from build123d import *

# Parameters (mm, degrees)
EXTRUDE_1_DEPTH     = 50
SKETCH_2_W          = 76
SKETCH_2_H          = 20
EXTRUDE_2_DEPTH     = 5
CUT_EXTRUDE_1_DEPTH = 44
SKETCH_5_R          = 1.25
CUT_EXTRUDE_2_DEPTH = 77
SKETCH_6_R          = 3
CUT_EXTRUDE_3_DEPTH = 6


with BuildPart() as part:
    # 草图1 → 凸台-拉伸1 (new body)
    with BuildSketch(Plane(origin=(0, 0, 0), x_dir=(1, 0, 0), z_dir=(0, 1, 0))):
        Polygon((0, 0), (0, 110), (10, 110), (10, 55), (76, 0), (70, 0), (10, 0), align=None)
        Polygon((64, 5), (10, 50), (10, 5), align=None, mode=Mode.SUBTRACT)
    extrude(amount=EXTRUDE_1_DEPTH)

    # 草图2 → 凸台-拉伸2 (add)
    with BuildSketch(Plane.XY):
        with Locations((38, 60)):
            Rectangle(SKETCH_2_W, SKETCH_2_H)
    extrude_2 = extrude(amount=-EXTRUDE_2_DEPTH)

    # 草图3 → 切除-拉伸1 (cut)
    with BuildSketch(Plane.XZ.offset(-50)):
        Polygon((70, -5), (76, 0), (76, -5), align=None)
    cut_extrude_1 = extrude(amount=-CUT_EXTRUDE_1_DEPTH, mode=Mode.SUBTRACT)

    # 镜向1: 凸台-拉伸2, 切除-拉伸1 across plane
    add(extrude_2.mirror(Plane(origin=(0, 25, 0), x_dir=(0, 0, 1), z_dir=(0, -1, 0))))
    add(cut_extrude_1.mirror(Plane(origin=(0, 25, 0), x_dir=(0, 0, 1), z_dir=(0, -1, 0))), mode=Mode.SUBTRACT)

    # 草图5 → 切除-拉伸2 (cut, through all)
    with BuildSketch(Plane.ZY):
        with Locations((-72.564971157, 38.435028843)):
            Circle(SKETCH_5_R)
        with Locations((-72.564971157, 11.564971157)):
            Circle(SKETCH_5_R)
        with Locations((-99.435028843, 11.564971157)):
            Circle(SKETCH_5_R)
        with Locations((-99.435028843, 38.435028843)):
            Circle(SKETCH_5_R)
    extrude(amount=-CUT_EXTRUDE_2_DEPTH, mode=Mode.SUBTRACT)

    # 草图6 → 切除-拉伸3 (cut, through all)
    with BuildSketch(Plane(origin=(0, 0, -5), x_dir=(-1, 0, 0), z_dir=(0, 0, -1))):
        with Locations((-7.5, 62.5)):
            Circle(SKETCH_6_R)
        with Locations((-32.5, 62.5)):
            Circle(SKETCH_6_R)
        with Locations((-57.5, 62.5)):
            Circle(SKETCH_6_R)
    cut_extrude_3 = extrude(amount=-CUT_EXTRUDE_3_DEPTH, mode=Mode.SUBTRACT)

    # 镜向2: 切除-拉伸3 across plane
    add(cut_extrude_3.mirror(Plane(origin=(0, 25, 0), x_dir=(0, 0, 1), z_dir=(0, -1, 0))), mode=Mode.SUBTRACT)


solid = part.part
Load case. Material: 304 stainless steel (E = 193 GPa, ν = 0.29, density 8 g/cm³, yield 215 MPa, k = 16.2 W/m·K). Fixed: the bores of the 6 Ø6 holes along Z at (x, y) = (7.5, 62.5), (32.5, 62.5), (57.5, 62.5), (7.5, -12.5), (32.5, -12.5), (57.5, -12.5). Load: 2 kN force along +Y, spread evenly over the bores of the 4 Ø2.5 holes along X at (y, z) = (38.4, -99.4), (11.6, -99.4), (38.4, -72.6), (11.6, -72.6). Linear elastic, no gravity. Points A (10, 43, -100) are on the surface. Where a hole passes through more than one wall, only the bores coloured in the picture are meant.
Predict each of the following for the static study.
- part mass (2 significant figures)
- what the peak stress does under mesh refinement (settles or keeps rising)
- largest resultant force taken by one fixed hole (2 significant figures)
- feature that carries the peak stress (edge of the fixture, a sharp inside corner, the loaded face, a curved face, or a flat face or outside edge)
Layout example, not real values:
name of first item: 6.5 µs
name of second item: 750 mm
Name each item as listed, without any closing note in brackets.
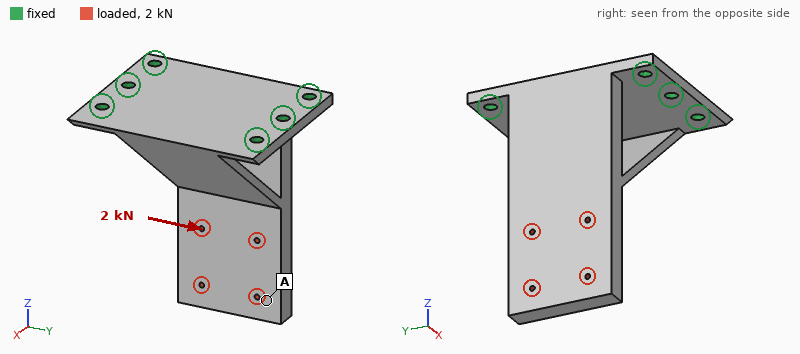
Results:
part mass: 790 g
what the peak stress does under mesh refinement: keeps rising
largest resultant force taken by one fixed hole: 2.2 kN
feature that carries the peak stress: edge of the fixture
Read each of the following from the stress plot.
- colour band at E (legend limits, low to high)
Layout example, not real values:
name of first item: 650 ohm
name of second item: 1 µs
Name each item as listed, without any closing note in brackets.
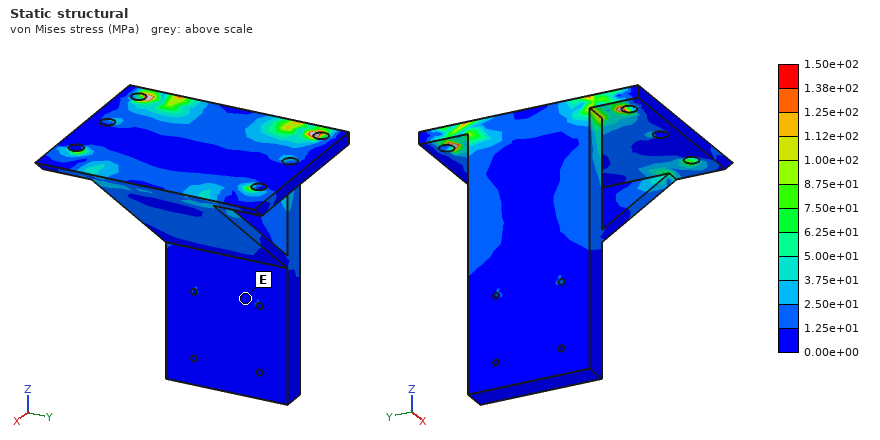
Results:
colour band at E: 0.00e+00 to 1.25e+01 MPa
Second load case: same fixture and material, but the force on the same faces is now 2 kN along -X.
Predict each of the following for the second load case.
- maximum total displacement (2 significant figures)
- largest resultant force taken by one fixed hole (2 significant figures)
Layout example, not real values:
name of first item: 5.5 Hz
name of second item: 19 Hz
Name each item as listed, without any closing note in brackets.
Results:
maximum total displacement: 0.24 mm
largest resultant force taken by one fixed hole: 1.7 kN
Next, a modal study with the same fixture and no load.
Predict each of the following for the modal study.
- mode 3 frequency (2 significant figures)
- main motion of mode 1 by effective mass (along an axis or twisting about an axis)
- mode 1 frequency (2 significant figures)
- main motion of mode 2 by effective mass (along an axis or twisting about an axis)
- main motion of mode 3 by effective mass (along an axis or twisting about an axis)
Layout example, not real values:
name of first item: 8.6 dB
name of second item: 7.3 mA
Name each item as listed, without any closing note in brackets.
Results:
mode 3 frequency: 2700 Hz
main motion of mode 1 by effective mass: along X
mode 1 frequency: 1200 Hz
main motion of mode 2 by effective mass: along Y
main motion of mode 3 by effective mass: along Z
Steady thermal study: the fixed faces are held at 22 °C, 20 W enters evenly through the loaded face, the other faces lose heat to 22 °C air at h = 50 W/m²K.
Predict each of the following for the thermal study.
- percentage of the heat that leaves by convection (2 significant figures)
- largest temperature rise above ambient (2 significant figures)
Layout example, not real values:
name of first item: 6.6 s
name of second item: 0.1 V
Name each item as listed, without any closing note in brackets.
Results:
percentage of the heat that leaves by convection: 95 %
largest temperature rise above ambient: 54 K
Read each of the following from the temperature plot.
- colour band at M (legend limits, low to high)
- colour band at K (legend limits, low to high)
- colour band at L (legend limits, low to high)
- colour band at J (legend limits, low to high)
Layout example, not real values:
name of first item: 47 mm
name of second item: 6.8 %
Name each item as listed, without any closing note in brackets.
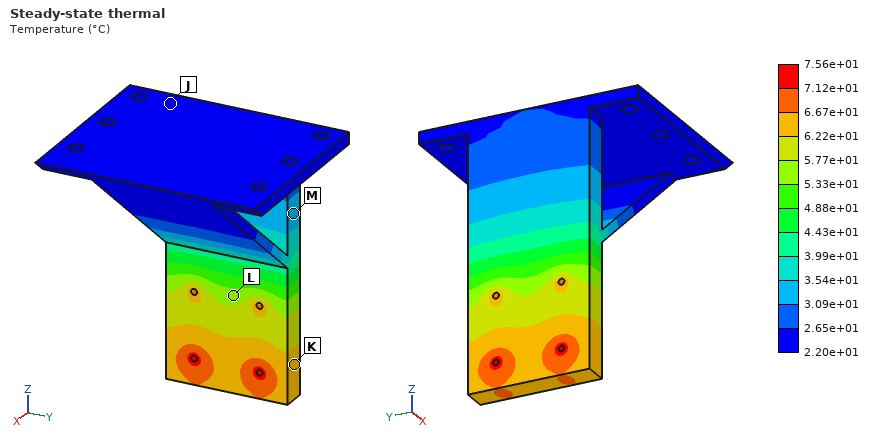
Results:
colour band at M: 3.09e+01 to 3.54e+01 °C
colour band at K: 6.22e+01 to 6.67e+01 °C
colour band at L: 5.33e+01 to 5.77e+01 °C
colour band at J: 2.20e+01 to 2.65e+01 °C
